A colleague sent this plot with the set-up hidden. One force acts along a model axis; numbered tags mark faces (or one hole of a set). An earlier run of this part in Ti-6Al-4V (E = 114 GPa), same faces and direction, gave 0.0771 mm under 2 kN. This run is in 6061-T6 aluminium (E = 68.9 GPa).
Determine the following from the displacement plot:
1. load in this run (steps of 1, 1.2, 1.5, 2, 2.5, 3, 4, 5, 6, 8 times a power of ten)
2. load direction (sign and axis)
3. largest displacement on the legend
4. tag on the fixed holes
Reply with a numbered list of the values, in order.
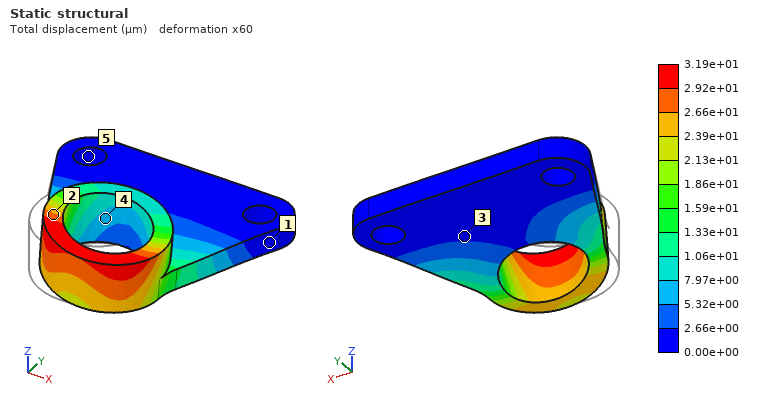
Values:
1. 500 N
2. +X
3. 3.19e+01 µm
4. 5
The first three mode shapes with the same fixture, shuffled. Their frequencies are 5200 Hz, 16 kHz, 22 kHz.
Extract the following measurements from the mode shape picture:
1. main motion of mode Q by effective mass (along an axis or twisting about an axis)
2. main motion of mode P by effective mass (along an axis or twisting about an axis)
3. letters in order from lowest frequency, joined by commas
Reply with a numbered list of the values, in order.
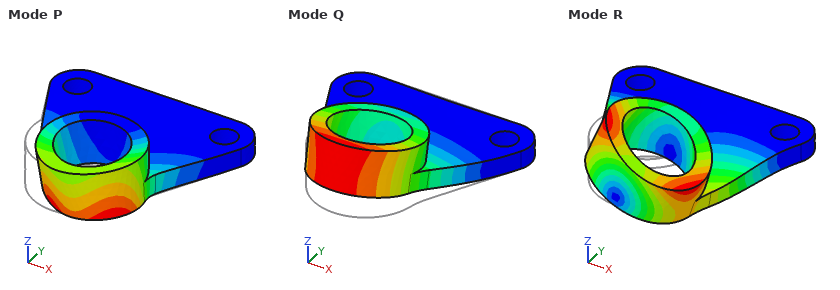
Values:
1. along Z
2. along X
3. Q, R, P
